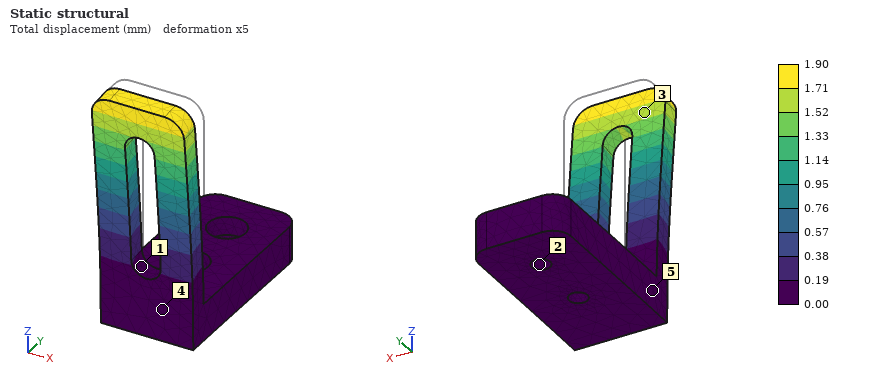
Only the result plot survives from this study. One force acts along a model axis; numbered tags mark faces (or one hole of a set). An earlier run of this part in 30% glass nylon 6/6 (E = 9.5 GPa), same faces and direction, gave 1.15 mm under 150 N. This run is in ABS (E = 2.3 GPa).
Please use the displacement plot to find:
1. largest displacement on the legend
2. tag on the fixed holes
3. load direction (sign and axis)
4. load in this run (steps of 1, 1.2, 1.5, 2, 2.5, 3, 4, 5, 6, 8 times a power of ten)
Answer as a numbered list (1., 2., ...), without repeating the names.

1. 1.90 mm
2. 2
3. -Y
4. 60 N
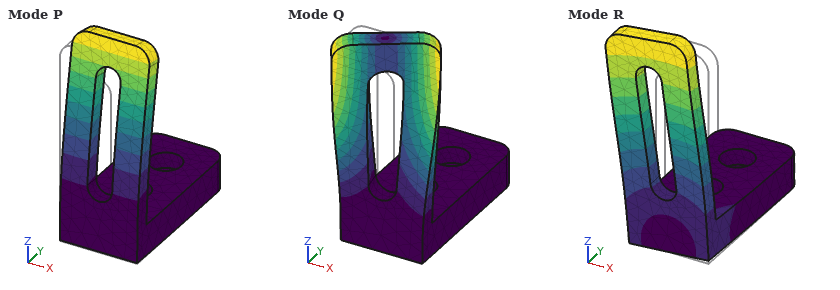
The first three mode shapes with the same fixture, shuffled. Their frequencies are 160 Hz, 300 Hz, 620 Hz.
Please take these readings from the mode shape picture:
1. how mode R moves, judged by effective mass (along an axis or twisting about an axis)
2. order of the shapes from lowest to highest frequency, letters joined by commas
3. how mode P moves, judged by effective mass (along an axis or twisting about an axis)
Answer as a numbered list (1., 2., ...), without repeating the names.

1. along X
2. P, R, Q
3. along Y
